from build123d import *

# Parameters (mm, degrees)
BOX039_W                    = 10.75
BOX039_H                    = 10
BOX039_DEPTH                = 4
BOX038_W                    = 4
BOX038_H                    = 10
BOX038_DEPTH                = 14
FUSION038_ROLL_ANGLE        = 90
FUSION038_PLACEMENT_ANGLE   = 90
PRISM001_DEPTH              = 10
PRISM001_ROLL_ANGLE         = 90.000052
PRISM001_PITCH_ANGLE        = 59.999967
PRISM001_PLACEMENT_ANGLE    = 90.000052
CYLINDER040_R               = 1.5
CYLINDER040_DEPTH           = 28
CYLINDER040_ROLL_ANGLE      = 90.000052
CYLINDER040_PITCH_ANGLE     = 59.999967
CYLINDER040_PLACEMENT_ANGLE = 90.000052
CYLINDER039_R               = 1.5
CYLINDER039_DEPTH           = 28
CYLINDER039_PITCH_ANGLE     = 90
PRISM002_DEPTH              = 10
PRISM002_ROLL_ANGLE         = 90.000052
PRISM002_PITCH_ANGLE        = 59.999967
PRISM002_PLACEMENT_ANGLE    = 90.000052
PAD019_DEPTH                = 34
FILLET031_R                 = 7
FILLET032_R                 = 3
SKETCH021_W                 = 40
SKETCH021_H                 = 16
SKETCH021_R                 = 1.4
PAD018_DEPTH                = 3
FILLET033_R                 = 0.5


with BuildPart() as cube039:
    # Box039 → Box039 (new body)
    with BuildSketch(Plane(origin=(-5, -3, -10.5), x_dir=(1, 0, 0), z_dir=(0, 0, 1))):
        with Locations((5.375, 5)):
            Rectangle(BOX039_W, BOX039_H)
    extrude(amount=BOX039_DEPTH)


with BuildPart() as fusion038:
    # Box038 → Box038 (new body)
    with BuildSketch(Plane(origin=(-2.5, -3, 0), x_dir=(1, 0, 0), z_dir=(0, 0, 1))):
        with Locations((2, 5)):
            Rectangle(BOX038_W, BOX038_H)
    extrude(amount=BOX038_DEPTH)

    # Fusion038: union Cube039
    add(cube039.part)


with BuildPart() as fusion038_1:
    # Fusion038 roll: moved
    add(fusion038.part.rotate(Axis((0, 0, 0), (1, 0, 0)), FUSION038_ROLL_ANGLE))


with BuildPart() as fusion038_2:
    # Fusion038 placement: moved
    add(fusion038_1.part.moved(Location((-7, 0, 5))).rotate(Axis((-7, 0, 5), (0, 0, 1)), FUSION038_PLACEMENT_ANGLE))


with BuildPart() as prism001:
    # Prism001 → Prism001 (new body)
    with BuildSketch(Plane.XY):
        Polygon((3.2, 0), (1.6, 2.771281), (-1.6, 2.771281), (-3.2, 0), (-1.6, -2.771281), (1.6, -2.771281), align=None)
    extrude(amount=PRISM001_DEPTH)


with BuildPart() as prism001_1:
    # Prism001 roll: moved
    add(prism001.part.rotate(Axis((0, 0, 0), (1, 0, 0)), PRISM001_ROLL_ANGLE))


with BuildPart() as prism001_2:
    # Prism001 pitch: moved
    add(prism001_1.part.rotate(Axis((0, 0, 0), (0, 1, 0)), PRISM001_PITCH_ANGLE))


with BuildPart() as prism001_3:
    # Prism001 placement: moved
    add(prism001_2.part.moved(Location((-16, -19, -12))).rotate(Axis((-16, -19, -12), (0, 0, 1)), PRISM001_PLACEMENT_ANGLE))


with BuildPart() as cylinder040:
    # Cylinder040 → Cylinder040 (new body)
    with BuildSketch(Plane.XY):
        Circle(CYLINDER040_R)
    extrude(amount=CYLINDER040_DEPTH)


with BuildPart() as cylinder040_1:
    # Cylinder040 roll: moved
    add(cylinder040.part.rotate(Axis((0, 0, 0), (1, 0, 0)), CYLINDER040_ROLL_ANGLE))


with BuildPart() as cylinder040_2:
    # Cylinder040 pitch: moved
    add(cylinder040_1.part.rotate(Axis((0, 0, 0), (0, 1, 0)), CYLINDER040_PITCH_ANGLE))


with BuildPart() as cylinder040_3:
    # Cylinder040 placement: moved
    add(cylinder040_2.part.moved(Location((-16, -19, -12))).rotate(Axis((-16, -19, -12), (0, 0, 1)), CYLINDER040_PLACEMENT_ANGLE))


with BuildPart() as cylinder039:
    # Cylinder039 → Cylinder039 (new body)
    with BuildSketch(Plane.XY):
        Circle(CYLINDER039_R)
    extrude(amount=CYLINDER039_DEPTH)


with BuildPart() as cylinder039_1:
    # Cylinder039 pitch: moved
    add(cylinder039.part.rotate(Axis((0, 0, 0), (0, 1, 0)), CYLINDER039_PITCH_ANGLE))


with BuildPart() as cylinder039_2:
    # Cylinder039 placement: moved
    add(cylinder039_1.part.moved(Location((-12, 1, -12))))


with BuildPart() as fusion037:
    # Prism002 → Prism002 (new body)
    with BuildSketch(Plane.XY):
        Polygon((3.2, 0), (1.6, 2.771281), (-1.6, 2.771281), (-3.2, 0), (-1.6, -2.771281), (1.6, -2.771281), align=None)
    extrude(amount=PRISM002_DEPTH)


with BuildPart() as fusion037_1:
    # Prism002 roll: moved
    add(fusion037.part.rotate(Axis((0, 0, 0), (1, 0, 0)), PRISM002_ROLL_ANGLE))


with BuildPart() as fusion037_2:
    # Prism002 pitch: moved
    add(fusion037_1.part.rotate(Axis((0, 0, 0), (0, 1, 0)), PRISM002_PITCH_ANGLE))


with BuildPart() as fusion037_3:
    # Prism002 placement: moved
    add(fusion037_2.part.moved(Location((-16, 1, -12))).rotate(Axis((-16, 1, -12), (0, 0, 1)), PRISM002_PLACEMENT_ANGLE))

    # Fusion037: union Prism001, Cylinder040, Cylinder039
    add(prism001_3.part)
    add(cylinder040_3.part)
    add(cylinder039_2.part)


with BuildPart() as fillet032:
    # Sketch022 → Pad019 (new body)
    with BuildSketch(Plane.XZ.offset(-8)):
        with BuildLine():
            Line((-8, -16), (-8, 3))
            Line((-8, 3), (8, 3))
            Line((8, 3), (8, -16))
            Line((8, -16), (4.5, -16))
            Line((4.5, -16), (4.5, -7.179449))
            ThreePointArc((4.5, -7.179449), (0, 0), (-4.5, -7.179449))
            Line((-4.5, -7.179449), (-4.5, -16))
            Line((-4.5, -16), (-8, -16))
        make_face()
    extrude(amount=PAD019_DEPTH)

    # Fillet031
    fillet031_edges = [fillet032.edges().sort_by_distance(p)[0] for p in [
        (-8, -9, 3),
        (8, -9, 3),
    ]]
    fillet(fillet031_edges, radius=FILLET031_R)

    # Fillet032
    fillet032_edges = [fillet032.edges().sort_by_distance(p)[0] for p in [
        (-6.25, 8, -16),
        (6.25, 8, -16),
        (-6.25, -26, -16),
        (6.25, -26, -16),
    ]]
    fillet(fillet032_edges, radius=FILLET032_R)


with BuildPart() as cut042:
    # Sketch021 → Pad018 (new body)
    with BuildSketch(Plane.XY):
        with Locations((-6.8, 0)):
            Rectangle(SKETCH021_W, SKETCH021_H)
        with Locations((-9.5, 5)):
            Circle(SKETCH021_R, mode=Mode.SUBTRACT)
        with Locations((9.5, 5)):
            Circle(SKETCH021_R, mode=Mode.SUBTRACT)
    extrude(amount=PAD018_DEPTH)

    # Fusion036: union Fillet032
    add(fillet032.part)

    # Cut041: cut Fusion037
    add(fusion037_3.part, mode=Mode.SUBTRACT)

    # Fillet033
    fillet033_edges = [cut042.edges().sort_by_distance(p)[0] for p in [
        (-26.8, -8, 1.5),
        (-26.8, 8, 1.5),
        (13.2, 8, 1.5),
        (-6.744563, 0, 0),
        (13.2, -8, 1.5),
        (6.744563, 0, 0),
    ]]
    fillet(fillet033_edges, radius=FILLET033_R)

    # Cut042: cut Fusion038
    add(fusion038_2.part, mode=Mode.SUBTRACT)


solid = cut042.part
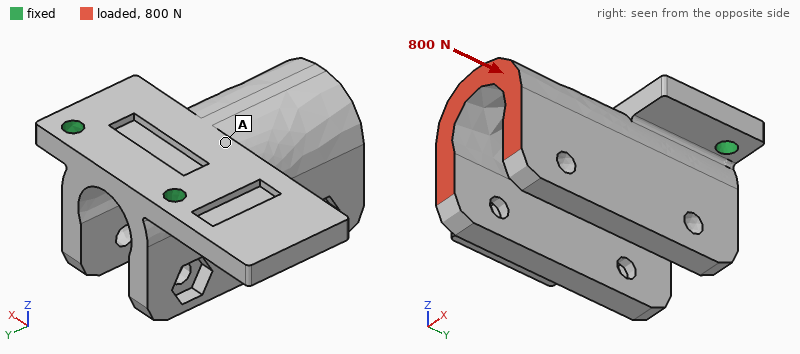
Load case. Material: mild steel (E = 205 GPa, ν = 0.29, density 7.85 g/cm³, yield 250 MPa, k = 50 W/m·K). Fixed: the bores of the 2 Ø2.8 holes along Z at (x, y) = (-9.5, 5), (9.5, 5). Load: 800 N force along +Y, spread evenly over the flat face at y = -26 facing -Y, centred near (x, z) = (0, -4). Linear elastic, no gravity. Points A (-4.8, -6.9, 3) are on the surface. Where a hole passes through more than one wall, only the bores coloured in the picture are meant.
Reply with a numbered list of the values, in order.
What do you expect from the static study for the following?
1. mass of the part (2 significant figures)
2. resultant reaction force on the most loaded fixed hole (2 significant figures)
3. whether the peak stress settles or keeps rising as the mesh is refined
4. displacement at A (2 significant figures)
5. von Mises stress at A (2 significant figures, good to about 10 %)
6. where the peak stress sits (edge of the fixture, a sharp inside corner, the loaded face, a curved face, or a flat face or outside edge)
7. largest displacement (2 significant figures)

1. 47 g
2. 410 N
3. keeps rising
4. 12 µm
5. 18 MPa
6. edge of the fixture
7. 37 µm
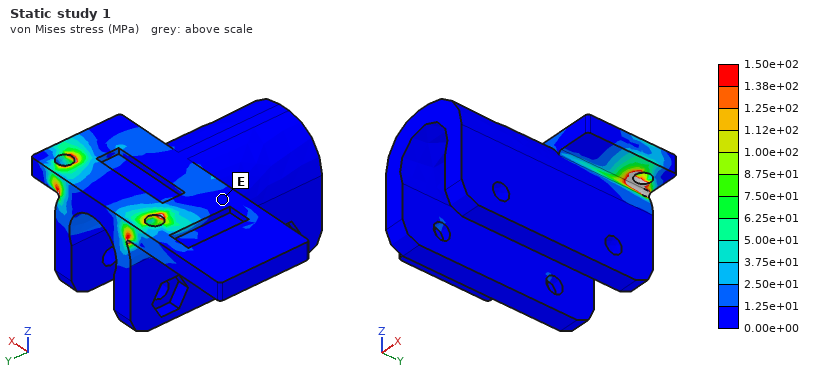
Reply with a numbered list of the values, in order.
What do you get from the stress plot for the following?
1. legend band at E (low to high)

1. 0.00e+00 to 1.25e+01 MPa
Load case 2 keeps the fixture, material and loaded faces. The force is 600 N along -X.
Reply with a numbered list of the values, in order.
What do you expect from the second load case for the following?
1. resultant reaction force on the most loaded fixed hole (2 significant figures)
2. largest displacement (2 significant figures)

1. 1.0 kN
2. 51 µm
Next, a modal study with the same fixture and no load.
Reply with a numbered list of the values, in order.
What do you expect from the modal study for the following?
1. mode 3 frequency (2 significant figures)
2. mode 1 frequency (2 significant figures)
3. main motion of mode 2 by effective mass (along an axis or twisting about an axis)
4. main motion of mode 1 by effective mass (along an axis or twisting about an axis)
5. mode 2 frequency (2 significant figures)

1. 6400 Hz
2. 2800 Hz
3. along X
4. along Z
5. 4900 Hz
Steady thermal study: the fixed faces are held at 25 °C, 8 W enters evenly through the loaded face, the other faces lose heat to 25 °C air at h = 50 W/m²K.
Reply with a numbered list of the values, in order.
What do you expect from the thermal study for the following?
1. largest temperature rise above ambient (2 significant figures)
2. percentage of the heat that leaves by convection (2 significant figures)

1. 34 K
2. 39 %
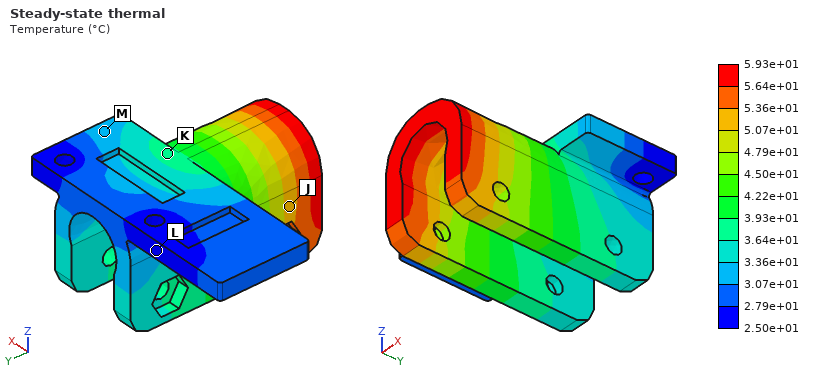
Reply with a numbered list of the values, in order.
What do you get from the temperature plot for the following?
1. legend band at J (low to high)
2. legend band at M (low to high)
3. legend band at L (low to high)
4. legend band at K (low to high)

1. 5.07e+01 to 5.36e+01 °C
2. 3.07e+01 to 3.36e+01 °C
3. 2.50e+01 to 2.79e+01 °C
4. 3.64e+01 to 3.93e+01 °C
